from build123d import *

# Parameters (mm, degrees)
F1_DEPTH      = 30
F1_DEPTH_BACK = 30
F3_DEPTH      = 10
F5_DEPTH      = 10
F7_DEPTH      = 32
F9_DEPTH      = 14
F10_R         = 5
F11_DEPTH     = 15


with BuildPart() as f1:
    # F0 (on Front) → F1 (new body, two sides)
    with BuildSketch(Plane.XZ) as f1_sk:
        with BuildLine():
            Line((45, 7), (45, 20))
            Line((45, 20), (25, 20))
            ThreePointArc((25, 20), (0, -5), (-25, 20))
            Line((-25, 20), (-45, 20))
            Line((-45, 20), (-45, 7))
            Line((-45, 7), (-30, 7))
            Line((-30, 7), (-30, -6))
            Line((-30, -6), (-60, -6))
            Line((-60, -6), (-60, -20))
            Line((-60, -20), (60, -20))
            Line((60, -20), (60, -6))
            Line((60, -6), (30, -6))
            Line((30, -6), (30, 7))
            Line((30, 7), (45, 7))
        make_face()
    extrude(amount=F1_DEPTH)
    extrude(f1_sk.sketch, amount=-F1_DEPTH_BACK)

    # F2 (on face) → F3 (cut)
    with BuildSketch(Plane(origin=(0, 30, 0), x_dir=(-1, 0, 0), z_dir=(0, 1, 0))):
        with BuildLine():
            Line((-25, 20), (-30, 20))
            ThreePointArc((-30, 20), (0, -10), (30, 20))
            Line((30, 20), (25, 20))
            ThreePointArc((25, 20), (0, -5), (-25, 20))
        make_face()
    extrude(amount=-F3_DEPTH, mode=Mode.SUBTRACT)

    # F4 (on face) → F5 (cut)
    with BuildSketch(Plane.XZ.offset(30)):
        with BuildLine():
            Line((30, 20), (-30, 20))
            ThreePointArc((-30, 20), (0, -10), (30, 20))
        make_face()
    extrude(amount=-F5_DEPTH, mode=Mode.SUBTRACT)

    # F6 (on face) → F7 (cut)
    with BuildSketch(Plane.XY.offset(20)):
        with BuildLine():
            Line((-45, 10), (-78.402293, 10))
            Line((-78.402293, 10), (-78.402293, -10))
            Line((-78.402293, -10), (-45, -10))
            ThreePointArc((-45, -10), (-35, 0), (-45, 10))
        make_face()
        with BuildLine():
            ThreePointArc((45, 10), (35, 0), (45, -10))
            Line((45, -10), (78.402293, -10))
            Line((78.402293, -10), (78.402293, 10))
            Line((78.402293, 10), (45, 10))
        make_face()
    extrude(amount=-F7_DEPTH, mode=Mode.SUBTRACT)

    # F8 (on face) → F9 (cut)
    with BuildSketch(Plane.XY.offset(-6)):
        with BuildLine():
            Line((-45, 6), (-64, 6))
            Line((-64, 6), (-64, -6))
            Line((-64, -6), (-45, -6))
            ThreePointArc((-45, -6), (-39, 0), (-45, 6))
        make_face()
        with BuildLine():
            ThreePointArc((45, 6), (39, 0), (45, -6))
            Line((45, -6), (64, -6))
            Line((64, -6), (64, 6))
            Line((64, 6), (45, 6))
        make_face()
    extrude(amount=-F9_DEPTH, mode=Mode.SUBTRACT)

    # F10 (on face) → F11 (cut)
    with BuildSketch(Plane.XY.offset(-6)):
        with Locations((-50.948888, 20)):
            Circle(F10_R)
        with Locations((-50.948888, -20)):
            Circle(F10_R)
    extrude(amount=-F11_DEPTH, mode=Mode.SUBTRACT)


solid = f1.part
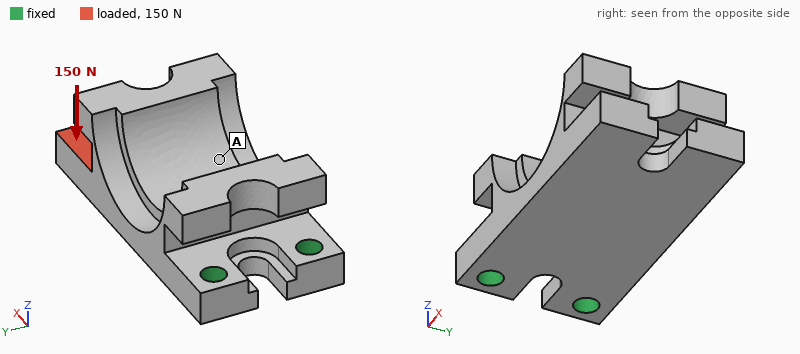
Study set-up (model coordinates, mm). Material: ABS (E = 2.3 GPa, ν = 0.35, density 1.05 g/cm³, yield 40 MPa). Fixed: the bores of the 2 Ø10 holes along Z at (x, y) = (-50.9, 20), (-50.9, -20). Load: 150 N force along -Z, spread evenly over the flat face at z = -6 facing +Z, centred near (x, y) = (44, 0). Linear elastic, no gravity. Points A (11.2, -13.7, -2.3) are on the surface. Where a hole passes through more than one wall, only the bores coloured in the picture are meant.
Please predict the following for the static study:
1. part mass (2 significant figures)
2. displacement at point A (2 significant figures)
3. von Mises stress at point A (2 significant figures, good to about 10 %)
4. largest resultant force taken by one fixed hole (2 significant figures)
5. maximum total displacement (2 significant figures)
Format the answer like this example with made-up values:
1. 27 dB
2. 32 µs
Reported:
1. 140 g
2. 0.67 mm
3. 1.8 MPa
4. 76 N
5. 1.5 mm
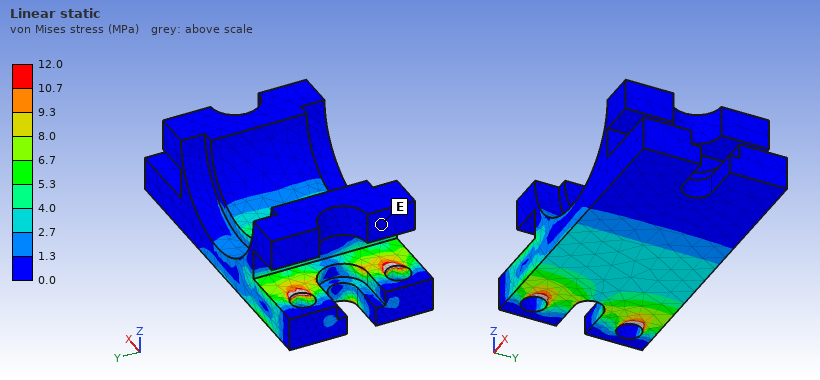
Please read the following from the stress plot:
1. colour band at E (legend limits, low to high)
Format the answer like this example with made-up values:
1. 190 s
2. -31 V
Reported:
1. 0.0 to 1.3 MPa
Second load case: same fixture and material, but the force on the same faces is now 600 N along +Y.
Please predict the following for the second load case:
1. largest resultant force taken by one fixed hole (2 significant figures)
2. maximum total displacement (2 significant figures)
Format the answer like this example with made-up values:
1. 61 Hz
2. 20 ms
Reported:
1. 1.3 kN
2. 0.55 mm
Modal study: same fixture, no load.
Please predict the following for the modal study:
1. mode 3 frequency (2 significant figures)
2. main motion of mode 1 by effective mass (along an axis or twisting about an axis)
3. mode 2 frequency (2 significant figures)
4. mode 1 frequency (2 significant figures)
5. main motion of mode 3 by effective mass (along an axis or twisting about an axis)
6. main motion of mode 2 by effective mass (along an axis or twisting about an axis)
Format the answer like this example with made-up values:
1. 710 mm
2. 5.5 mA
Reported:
1. 950 Hz
2. along Z
3. 780 Hz
4. 240 Hz
5. along Y
6. along Y
